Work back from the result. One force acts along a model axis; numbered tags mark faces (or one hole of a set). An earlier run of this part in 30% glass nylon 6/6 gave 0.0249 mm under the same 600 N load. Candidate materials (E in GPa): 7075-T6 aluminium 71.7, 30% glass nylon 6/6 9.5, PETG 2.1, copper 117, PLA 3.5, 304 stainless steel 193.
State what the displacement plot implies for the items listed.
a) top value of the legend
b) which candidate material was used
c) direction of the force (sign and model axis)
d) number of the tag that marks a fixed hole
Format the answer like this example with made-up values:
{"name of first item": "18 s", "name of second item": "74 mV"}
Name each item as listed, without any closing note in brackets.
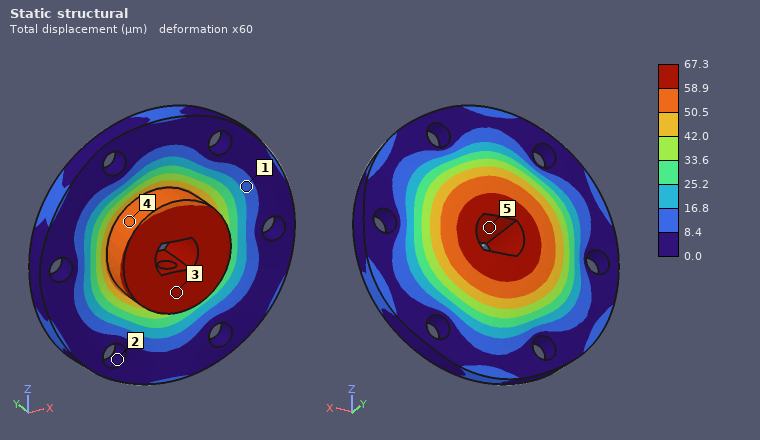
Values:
{"top value of the legend": "67.3 µm", "which candidate material was used": "PLA", "direction of the force": "+Y", "number of the tag that marks a fixed hole": "2"}
